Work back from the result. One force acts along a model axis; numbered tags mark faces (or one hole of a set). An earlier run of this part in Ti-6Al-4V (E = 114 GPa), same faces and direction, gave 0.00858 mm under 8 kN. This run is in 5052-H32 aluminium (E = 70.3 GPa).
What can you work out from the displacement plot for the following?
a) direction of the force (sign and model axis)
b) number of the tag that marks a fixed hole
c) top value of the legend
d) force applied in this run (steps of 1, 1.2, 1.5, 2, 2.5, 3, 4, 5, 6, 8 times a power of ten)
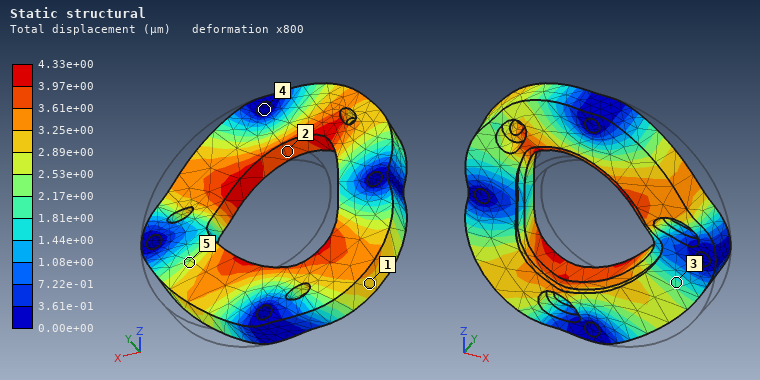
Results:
-X
4
4.33e+00 µm
2.5 kN
